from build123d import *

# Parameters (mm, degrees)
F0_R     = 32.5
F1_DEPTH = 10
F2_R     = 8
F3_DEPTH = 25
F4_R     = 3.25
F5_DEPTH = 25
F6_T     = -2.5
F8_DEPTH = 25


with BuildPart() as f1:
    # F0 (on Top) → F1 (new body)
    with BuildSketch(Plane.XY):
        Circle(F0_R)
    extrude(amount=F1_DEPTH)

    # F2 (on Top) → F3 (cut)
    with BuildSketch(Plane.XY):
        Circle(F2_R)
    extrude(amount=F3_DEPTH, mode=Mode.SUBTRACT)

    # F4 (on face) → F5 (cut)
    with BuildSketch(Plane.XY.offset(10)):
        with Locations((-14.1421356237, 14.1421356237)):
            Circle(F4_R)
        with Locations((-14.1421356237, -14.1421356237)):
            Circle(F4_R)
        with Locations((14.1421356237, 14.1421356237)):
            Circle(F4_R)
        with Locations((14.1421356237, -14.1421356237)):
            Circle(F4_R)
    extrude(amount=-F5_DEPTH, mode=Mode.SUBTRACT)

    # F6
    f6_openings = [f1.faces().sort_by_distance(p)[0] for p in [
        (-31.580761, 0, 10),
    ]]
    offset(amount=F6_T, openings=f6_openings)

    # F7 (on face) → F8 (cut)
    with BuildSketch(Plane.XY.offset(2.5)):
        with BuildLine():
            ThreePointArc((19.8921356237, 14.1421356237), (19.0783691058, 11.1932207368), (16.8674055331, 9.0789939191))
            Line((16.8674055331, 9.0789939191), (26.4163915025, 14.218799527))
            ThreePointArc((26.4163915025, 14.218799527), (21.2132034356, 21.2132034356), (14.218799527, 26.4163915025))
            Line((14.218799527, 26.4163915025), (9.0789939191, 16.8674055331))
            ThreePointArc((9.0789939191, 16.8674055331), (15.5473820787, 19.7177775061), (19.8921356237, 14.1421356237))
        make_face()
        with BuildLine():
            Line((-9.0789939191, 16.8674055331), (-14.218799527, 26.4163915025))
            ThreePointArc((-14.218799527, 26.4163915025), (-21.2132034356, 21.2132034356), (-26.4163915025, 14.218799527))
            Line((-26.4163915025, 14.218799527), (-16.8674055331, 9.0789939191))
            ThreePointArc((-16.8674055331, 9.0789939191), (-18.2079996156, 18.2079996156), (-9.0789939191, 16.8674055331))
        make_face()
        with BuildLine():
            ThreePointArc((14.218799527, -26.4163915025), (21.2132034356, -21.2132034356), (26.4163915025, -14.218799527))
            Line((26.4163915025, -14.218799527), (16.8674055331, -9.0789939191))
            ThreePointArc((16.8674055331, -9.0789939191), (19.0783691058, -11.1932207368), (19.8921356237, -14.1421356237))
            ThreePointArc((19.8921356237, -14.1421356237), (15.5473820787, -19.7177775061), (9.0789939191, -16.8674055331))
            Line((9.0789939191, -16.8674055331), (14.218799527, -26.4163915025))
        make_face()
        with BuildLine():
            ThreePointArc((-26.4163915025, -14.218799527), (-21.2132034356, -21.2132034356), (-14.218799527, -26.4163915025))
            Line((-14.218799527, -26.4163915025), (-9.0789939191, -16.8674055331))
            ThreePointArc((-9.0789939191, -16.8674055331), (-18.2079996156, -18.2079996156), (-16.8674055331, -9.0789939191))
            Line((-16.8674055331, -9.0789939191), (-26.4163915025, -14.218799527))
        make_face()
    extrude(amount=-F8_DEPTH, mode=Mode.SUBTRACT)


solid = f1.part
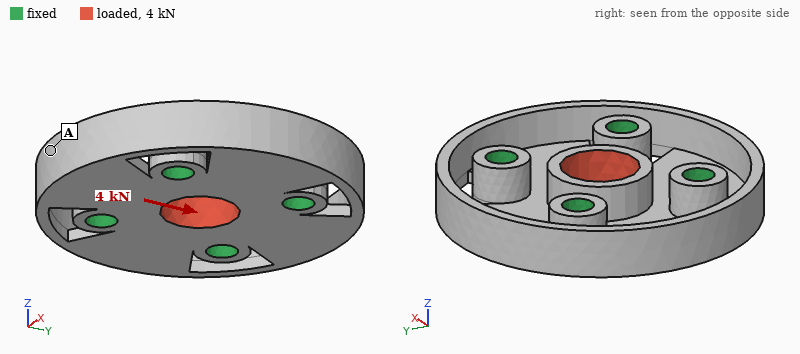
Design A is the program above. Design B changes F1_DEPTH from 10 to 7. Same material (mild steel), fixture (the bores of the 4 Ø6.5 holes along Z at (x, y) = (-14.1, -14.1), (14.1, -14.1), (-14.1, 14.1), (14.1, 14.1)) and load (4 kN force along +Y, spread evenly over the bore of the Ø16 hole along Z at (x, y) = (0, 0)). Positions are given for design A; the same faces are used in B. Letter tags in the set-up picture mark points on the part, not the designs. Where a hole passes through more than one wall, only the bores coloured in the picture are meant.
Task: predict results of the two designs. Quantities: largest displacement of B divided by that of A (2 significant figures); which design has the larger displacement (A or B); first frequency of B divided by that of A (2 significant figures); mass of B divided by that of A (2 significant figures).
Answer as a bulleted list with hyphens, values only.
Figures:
- 0.63
- A
- 1.1
- 0.79
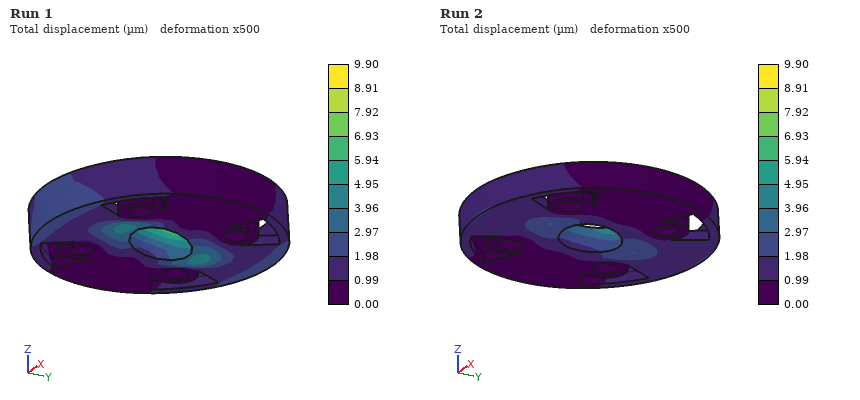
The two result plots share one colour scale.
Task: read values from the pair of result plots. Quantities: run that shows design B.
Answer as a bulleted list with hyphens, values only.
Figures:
- Run 2
